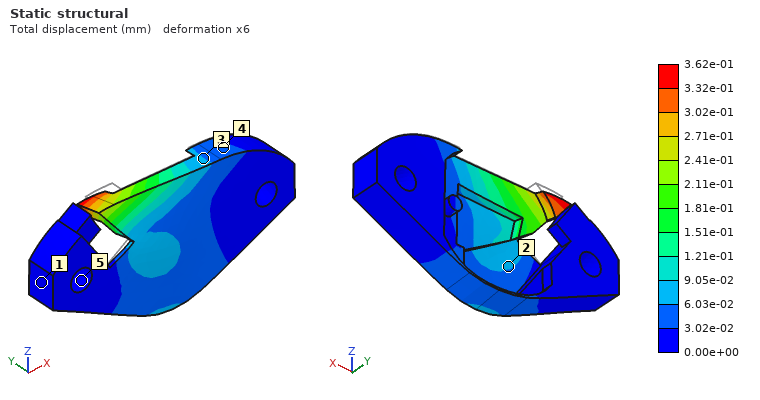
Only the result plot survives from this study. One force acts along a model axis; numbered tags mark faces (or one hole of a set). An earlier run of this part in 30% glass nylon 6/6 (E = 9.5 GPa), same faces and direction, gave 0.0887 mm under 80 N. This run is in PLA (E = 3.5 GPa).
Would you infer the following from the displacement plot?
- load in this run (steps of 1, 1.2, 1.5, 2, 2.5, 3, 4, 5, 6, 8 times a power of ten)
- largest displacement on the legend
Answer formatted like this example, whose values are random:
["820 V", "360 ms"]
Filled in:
["120 N", "3.62e-01 mm"]
